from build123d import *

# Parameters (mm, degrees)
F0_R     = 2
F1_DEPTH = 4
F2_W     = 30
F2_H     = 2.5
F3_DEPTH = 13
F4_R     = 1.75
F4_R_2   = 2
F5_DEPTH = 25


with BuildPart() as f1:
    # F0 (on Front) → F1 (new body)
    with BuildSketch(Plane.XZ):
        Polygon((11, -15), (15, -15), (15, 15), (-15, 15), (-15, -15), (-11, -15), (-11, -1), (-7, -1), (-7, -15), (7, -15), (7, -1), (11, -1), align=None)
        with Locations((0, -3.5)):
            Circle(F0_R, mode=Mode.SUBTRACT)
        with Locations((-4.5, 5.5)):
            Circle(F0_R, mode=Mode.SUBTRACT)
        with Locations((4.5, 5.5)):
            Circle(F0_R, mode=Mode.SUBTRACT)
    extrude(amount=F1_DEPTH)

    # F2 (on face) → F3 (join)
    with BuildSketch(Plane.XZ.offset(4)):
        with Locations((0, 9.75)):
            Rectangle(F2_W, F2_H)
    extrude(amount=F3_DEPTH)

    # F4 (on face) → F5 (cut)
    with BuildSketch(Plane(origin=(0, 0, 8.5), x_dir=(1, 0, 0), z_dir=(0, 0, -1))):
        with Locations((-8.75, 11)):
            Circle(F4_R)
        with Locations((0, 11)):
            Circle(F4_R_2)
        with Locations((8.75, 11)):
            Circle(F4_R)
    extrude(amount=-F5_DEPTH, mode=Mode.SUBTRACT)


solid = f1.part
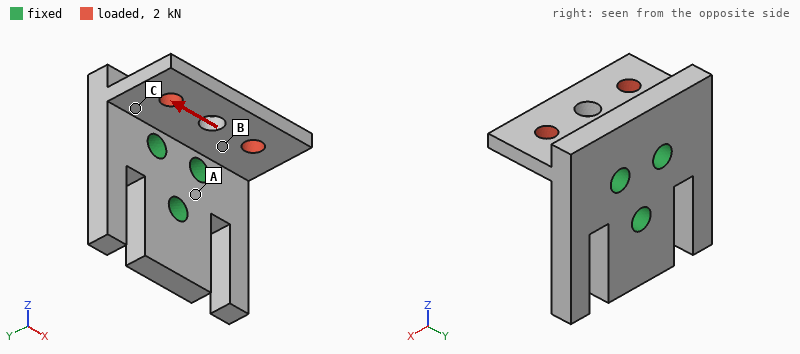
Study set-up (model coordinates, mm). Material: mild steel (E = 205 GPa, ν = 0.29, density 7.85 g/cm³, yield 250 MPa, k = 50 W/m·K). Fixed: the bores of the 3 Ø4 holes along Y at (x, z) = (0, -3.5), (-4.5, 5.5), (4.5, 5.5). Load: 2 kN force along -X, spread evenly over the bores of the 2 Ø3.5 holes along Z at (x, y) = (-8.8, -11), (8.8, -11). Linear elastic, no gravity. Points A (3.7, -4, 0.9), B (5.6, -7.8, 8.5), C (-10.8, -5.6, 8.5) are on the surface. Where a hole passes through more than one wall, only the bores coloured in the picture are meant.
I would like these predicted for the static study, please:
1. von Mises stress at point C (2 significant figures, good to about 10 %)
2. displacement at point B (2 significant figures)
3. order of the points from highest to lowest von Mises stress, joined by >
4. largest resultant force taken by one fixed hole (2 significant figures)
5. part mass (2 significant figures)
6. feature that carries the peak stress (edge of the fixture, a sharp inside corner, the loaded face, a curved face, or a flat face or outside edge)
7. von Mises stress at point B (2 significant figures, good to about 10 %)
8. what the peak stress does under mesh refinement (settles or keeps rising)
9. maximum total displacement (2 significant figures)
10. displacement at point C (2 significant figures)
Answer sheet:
44 MPa
7.1 µm
B > C > A
1.7 kN
31 g
edge of the fixture
79 MPa
keeps rising
19 µm
7.3 µm
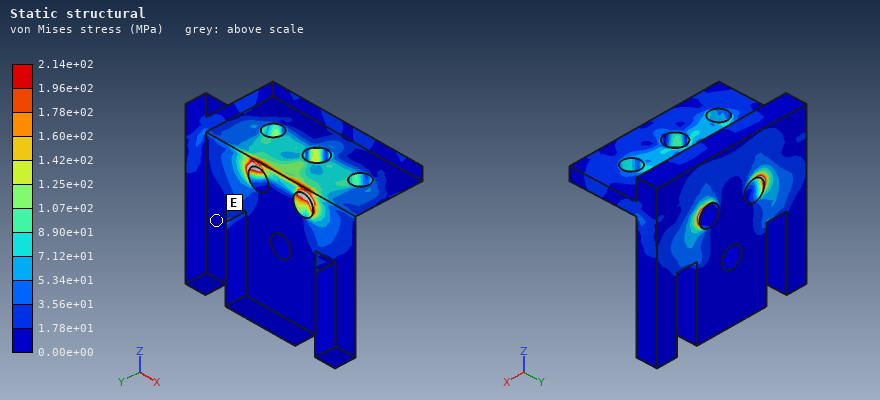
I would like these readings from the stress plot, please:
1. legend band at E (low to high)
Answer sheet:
0.00e+00 to 1.78e+01 MPa
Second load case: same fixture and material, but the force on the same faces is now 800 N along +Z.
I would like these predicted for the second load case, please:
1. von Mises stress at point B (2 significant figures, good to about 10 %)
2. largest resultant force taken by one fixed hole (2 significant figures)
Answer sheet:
83 MPa
370 N
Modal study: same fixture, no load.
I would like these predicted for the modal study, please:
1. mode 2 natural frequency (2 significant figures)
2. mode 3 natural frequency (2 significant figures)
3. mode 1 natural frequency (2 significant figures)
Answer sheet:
8700 Hz
9600 Hz
8500 Hz
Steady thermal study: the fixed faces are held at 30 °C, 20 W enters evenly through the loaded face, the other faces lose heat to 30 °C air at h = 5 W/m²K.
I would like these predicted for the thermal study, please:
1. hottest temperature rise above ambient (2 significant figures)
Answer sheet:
74 K
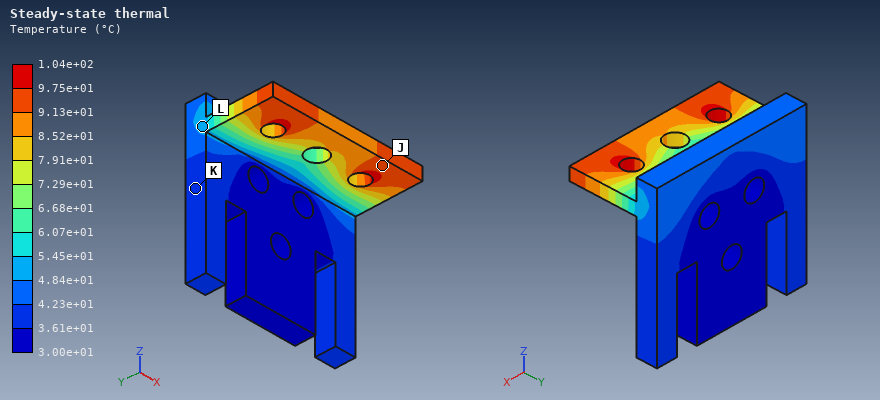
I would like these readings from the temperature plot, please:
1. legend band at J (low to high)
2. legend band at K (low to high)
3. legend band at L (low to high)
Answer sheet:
9.13e+01 to 9.75e+01 °C
3.61e+01 to 4.23e+01 °C
4.84e+01 to 5.45e+01 °C
